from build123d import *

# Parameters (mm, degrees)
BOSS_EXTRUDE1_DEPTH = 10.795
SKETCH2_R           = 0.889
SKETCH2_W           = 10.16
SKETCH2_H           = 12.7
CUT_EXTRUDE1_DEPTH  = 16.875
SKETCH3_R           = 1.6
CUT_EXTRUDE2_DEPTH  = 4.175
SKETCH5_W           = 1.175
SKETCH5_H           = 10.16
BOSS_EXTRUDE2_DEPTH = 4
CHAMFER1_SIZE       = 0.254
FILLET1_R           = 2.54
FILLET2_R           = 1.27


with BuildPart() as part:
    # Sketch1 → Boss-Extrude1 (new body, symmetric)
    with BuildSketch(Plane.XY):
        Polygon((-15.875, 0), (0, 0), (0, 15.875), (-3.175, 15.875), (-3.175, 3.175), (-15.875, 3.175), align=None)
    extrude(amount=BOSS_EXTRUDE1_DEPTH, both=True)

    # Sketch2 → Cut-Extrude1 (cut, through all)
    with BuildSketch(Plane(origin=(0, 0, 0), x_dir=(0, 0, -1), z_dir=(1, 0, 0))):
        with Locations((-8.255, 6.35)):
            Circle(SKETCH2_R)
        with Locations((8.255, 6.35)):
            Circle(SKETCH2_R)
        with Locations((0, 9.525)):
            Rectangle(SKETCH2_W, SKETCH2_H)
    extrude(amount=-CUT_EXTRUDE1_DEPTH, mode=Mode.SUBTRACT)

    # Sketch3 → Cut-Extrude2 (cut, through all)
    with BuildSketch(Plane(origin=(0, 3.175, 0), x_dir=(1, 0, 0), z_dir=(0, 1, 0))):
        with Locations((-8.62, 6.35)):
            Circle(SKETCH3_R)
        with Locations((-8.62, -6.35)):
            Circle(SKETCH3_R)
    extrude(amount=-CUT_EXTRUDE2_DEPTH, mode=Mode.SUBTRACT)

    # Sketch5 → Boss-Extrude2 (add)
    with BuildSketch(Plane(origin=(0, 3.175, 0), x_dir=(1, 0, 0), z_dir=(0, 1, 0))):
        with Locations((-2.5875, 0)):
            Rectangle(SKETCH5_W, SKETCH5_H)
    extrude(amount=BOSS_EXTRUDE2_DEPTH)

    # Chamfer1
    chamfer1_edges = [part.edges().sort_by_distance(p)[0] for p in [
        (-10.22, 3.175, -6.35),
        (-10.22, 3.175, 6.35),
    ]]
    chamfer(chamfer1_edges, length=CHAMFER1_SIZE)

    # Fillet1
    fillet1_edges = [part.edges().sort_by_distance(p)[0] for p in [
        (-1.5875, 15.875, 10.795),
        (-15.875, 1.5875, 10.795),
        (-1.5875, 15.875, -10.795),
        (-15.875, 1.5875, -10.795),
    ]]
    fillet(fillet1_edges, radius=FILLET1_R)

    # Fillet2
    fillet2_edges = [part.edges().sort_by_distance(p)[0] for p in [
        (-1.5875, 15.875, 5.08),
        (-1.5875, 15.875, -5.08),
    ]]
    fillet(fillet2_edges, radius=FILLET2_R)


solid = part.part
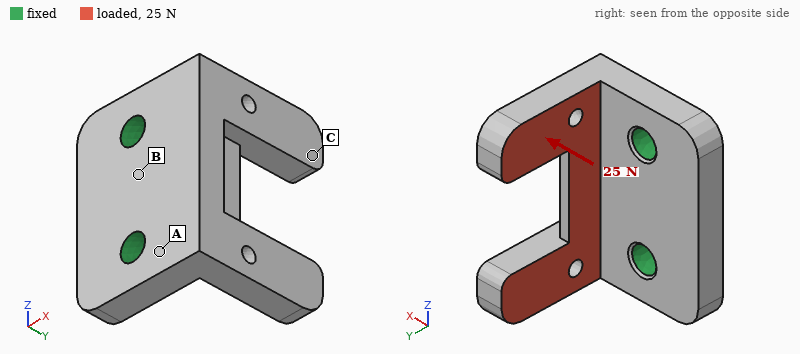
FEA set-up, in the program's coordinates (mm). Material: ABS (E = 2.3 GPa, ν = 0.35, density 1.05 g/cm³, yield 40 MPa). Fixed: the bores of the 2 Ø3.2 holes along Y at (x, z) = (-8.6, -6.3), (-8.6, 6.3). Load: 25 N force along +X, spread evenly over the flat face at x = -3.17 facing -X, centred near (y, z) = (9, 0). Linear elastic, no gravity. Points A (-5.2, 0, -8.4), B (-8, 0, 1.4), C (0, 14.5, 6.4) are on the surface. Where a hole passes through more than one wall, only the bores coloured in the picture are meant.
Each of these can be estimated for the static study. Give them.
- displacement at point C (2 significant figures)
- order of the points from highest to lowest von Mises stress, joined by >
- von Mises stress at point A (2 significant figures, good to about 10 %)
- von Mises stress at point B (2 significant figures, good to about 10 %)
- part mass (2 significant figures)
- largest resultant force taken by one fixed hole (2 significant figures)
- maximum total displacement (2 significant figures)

0.20 mm
A > B > C
4.5 MPa
2.0 MPa
1.6 g
13 N
0.23 mm
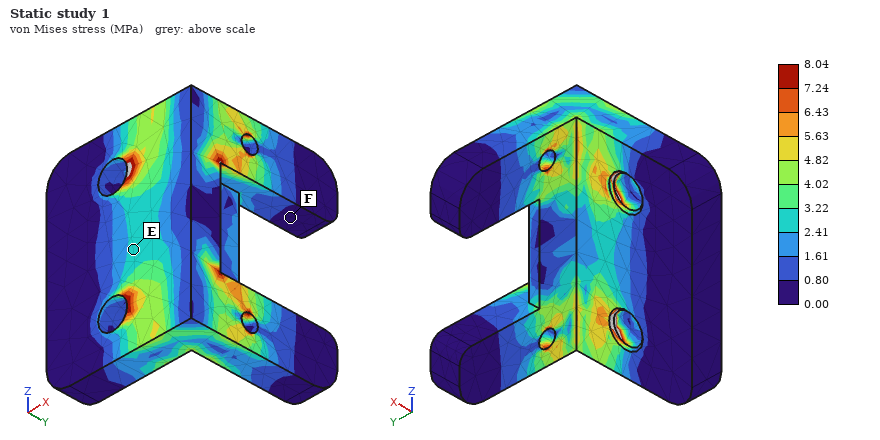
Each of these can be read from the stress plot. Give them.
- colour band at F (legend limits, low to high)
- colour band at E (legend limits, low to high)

0.00 to 0.80 MPa
2.41 to 3.22 MPa
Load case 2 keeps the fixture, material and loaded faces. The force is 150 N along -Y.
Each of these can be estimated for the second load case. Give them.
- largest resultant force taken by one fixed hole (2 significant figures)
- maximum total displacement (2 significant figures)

75 N
0.12 mm
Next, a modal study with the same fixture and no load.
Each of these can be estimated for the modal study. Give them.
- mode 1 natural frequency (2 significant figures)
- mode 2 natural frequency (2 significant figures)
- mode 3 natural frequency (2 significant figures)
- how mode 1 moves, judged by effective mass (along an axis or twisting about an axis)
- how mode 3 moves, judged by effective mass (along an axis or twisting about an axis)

2700 Hz
2900 Hz
5100 Hz
along X
along Z
